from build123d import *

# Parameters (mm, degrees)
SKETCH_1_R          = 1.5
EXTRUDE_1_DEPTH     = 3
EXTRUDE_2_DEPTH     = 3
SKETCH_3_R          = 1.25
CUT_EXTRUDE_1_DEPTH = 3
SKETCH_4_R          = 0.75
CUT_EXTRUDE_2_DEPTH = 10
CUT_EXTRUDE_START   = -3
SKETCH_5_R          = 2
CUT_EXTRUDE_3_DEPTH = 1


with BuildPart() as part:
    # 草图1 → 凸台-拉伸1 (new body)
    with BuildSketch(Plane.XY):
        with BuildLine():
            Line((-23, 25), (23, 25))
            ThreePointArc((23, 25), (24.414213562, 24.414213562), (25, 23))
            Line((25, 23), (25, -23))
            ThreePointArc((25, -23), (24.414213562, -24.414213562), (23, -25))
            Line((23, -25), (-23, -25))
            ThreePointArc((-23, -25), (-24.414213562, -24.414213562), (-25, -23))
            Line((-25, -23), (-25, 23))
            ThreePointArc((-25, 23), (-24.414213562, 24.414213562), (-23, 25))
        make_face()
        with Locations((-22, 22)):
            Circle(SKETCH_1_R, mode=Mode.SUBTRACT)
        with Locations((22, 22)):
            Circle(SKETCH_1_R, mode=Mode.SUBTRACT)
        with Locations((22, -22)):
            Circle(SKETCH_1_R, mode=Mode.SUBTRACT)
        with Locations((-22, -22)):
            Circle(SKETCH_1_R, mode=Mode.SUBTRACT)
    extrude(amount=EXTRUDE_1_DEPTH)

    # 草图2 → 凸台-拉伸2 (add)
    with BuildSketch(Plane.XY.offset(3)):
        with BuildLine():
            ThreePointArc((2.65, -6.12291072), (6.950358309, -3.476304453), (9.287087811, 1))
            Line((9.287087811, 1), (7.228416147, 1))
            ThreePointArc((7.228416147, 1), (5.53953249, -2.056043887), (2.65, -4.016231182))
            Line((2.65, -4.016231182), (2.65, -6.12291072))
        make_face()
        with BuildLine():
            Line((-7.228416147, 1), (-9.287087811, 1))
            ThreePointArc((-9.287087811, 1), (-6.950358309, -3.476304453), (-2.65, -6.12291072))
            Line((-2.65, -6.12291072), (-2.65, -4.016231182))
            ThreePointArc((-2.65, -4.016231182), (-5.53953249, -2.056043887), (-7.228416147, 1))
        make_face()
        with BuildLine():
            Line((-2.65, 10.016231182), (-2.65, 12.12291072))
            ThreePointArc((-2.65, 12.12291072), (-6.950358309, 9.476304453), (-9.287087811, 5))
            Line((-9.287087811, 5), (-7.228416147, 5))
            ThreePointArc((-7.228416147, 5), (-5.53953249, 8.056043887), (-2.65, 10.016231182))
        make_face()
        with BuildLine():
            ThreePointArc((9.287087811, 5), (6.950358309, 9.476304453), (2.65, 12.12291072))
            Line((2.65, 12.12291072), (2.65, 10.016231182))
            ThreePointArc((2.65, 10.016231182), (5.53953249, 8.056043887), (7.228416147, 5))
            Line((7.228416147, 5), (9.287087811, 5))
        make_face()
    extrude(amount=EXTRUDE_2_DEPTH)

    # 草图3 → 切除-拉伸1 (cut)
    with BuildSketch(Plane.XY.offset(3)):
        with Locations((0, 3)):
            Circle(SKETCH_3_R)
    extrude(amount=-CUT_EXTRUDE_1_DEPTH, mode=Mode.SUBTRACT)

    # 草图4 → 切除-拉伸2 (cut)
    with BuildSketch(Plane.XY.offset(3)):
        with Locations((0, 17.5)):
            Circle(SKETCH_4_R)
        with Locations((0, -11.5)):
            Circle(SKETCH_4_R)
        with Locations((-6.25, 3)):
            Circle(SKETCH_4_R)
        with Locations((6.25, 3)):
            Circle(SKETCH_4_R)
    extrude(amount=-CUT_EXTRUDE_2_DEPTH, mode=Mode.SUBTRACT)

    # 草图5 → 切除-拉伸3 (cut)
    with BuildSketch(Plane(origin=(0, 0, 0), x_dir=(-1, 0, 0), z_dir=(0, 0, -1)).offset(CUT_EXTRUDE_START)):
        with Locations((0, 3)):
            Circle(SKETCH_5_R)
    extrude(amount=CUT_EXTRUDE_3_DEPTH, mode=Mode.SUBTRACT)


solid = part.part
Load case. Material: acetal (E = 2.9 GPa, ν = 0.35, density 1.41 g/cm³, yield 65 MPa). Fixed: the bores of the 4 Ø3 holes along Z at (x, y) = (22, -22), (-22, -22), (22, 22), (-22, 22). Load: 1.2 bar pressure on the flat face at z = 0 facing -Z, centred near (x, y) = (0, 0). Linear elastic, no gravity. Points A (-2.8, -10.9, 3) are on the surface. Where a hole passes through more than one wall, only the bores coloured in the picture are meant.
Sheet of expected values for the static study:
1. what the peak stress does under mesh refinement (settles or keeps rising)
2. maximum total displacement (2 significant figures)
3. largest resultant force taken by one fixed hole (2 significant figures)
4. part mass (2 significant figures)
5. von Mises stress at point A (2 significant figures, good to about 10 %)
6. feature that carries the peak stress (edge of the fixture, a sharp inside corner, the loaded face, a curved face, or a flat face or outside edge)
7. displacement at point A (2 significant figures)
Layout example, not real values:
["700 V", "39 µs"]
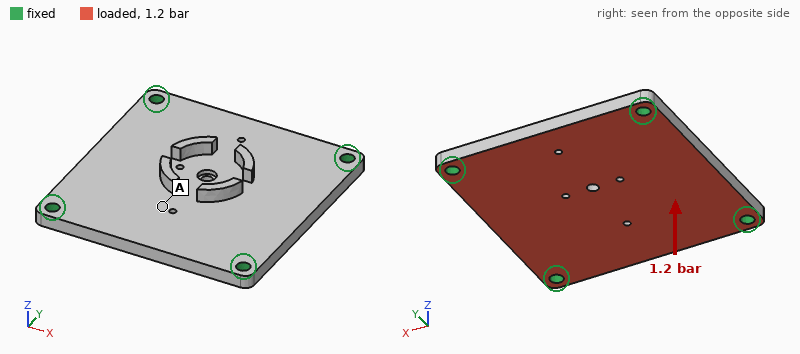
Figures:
["keeps rising", "0.49 mm", "74 N", "11 g", "7.6 MPa", "edge of the fixture", "0.41 mm"]
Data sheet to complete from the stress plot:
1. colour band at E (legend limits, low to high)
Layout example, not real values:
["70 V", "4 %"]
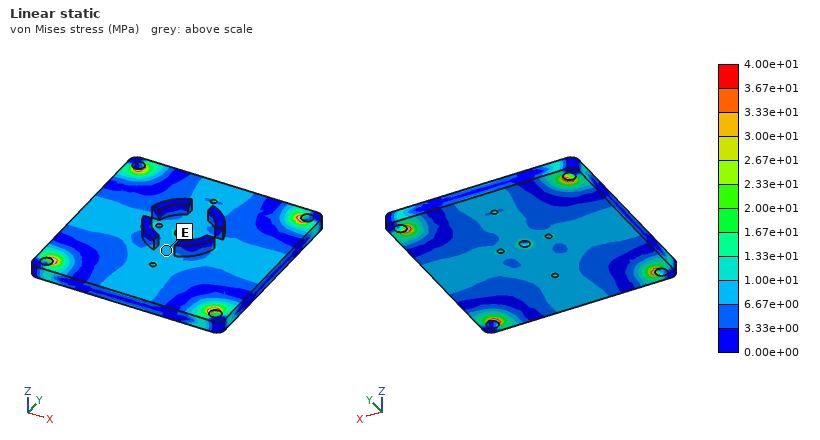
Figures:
["6.67e+00 to 1.00e+01 MPa"]
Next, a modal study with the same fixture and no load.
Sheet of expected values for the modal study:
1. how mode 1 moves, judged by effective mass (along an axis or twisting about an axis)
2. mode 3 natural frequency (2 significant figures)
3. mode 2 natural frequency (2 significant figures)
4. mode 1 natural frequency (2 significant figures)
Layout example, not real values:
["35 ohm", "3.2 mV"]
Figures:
["along Z", "2500 Hz", "2500 Hz", "1400 Hz"]
